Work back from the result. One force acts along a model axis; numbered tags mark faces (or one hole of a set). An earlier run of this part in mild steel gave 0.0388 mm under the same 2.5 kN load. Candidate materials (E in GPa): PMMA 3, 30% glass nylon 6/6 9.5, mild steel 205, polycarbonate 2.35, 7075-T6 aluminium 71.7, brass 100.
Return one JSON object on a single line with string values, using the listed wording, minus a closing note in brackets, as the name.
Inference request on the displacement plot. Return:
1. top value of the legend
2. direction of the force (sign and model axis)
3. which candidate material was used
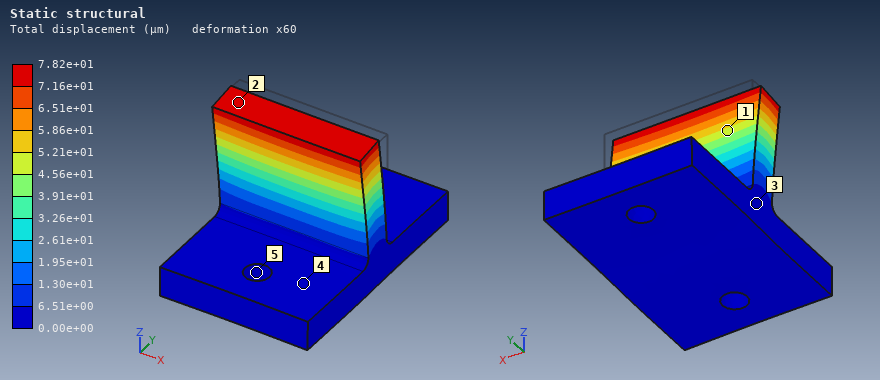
{"top value of the legend": "7.82e+01 µm", "direction of the force": "-Y", "which candidate material was used": "brass"}
